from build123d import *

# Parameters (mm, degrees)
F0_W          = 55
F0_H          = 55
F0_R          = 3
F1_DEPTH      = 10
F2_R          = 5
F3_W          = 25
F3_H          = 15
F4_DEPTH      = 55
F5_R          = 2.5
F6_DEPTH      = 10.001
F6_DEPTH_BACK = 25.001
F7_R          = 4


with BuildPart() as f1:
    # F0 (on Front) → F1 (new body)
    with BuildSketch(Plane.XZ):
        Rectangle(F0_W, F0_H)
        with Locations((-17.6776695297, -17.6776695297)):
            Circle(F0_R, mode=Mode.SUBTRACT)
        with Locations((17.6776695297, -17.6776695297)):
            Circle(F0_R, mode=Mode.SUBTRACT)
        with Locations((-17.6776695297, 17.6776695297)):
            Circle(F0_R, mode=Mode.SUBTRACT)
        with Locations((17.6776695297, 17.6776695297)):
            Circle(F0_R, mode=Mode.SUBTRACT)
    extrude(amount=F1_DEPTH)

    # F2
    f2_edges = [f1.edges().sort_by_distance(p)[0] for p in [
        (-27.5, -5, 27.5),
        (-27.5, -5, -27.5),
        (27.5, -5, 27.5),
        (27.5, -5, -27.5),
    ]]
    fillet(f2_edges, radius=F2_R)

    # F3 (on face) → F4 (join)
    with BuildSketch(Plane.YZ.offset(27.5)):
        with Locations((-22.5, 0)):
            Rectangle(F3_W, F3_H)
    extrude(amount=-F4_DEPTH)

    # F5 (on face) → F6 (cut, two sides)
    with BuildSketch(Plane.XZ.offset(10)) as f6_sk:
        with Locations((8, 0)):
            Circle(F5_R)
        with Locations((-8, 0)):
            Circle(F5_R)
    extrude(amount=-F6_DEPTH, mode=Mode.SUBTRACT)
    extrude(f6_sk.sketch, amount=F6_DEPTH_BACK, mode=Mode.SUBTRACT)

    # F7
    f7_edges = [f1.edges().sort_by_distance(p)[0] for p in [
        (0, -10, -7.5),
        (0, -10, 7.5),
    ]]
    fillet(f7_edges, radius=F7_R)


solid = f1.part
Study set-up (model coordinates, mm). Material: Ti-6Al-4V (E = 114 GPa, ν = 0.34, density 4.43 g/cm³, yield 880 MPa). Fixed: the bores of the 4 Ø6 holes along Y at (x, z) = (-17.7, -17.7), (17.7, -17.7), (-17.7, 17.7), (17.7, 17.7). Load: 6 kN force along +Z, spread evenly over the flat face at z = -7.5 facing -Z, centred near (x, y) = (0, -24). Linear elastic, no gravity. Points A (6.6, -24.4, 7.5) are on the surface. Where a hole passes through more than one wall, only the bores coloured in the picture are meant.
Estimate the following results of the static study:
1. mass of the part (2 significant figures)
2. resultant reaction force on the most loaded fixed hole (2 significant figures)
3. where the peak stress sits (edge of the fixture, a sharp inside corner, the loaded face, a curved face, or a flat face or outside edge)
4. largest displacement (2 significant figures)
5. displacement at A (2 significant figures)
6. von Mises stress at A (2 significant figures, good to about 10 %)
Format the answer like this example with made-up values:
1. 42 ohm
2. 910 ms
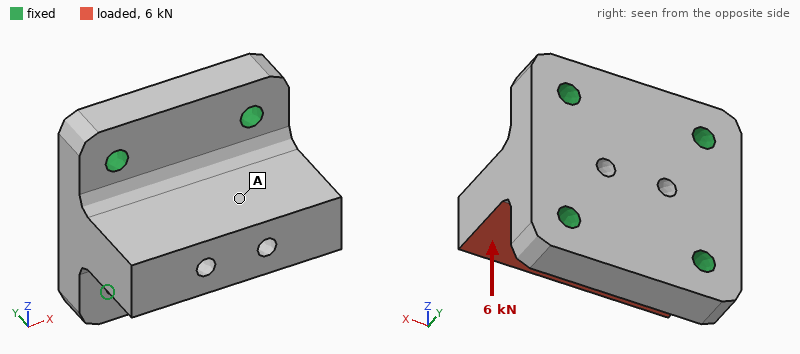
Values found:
1. 210 g
2. 2.5 kN
3. a curved face
4. 20 µm
5. 12 µm
6. 6.9 MPa
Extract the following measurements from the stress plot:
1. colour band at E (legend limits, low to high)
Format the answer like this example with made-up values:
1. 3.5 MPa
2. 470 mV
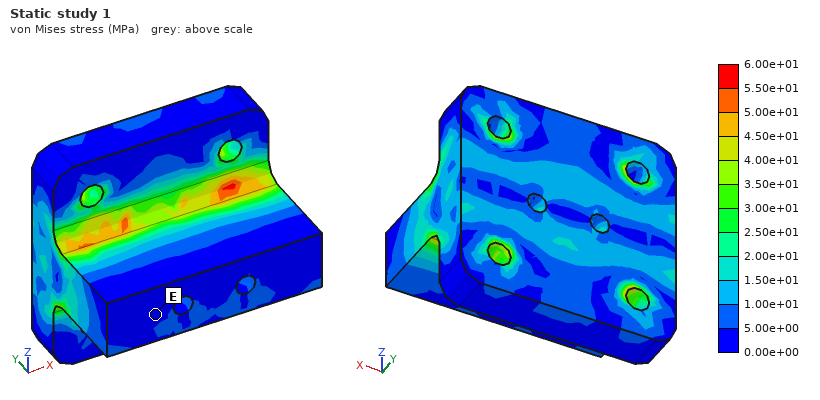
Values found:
1. 0.00e+00 to 5.00e+00 MPa
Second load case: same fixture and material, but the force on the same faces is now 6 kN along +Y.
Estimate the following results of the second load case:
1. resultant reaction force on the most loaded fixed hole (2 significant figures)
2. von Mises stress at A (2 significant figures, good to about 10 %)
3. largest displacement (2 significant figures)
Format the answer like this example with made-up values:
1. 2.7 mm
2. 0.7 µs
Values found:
1. 2.3 kN
2. 6.4 MPa
3. 13 µm
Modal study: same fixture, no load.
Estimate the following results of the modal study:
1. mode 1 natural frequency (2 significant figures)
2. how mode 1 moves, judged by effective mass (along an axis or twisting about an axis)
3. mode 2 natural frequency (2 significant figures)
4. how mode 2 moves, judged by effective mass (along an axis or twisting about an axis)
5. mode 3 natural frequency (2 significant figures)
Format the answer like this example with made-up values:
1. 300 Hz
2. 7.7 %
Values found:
1. 12 kHz
2. along Z
3. 13 kHz
4. along X
5. 17 kHz
